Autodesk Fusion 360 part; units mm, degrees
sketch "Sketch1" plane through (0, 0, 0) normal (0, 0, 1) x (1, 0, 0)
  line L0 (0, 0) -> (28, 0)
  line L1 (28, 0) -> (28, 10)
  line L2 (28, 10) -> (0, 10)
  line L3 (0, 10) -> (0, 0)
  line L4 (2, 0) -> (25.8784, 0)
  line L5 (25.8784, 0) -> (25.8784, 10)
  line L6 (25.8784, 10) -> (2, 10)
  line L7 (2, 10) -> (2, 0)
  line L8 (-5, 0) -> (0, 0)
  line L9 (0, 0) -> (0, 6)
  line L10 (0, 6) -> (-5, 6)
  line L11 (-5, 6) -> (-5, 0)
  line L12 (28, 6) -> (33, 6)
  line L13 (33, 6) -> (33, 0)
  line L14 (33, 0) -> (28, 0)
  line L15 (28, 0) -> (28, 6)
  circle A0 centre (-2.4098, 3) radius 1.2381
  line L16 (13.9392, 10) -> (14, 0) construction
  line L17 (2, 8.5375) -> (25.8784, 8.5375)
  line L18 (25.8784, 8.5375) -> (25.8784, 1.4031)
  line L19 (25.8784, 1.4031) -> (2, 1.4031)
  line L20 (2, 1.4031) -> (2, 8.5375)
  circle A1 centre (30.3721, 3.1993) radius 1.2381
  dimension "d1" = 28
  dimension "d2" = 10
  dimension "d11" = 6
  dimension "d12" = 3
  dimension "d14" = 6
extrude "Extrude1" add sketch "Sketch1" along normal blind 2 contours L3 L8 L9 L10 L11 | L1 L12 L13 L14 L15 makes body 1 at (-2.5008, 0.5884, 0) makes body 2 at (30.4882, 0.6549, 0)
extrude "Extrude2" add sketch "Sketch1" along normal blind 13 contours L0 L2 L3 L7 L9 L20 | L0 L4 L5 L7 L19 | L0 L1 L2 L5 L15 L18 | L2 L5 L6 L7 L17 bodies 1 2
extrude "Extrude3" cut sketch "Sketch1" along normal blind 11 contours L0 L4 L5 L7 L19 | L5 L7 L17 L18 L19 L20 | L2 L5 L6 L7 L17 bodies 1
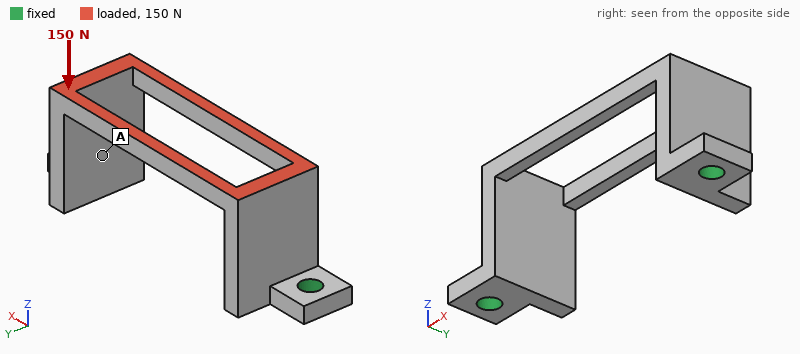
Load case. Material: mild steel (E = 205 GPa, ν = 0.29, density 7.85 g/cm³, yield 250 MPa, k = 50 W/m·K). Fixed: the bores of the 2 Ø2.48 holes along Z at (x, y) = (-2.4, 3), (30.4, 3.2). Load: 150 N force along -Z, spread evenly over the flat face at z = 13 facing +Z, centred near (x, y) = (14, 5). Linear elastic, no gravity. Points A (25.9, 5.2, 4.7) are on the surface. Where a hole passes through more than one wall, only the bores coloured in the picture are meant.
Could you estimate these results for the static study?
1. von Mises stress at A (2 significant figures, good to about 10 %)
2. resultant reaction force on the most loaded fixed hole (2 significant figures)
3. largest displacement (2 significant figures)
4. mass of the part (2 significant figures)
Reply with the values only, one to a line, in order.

9.7 MPa
81 N
17 µm
6.1 g
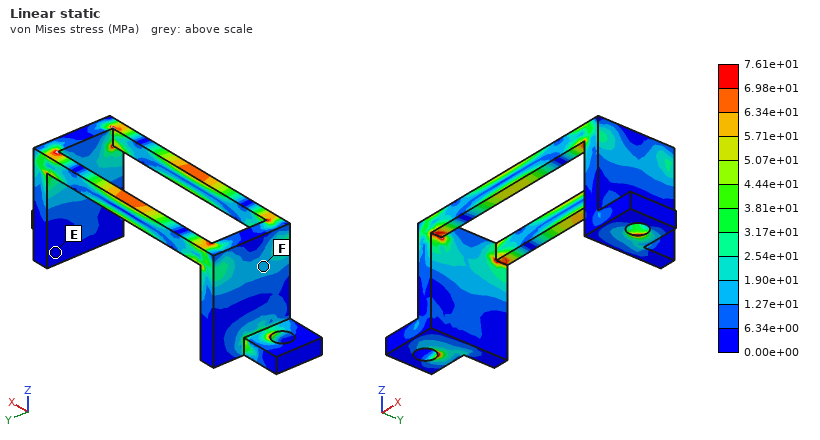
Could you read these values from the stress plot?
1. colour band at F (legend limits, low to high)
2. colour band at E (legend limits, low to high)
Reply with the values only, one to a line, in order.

1.27e+01 to 1.90e+01 MPa
0.00e+00 to 6.34e+00 MPa
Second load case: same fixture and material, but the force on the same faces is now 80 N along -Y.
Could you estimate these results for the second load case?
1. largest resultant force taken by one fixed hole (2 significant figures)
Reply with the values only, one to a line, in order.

40 N
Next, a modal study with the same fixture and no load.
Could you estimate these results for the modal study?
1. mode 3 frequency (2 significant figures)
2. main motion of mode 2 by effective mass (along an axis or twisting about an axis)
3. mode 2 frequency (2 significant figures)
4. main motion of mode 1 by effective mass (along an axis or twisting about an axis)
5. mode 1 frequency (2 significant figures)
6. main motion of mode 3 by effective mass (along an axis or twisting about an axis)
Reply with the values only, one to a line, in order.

9700 Hz
along Y
7500 Hz
along X
7000 Hz
twisting about Z
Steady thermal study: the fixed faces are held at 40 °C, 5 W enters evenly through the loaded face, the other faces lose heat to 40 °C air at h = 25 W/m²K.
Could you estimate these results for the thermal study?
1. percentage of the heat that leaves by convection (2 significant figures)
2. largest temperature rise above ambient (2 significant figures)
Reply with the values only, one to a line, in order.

14 %
66 K
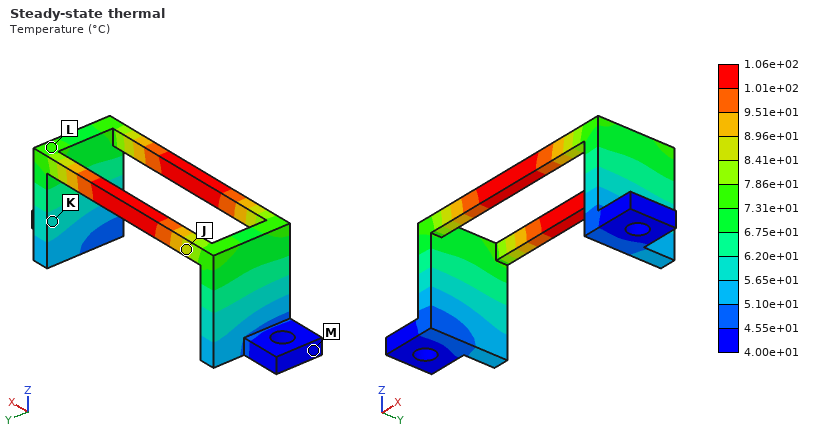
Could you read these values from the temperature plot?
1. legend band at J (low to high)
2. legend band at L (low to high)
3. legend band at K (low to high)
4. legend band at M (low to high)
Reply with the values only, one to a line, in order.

8.41e+01 to 8.96e+01 °C
7.31e+01 to 7.86e+01 °C
5.65e+01 to 6.20e+01 °C
4.00e+01 to 4.55e+01 °C
